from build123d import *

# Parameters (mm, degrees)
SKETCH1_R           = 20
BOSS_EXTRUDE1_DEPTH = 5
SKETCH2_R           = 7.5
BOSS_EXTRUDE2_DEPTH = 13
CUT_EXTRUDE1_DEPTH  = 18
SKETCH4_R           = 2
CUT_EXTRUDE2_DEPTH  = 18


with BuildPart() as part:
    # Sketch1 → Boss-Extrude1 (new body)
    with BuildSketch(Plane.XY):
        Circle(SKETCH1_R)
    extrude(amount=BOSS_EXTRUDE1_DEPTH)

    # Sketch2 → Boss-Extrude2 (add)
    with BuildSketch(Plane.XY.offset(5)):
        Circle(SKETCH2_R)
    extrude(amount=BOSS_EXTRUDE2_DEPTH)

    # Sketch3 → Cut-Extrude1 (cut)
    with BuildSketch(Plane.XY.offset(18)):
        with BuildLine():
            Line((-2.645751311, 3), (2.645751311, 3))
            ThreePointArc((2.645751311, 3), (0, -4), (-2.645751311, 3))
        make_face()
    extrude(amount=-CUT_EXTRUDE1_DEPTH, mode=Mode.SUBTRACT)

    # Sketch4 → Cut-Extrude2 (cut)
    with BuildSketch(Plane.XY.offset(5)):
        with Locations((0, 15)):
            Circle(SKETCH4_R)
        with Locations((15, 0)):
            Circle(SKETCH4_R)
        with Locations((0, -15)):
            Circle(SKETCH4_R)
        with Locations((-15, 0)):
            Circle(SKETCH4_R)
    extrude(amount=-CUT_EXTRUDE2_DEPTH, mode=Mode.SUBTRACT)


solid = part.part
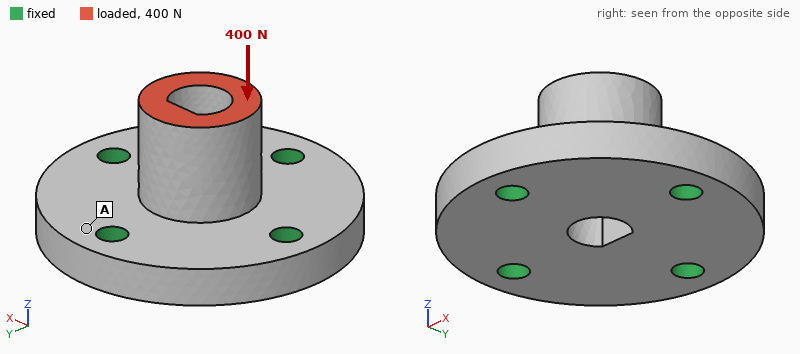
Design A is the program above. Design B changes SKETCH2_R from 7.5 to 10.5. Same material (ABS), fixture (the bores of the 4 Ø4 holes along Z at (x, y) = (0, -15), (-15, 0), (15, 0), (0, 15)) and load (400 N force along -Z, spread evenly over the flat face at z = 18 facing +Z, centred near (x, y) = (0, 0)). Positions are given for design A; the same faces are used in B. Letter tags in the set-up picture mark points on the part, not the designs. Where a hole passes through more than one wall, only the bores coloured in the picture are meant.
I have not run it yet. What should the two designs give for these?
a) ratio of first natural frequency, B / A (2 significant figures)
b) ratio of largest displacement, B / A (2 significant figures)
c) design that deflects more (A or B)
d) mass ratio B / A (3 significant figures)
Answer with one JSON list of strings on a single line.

["1.0", "0.46", "A", "1.29"]
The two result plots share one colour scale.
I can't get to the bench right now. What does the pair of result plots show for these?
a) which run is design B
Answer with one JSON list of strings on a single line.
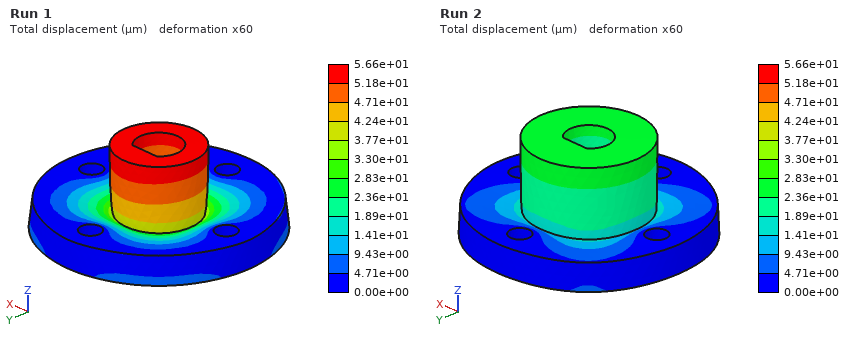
["Run 2"]
